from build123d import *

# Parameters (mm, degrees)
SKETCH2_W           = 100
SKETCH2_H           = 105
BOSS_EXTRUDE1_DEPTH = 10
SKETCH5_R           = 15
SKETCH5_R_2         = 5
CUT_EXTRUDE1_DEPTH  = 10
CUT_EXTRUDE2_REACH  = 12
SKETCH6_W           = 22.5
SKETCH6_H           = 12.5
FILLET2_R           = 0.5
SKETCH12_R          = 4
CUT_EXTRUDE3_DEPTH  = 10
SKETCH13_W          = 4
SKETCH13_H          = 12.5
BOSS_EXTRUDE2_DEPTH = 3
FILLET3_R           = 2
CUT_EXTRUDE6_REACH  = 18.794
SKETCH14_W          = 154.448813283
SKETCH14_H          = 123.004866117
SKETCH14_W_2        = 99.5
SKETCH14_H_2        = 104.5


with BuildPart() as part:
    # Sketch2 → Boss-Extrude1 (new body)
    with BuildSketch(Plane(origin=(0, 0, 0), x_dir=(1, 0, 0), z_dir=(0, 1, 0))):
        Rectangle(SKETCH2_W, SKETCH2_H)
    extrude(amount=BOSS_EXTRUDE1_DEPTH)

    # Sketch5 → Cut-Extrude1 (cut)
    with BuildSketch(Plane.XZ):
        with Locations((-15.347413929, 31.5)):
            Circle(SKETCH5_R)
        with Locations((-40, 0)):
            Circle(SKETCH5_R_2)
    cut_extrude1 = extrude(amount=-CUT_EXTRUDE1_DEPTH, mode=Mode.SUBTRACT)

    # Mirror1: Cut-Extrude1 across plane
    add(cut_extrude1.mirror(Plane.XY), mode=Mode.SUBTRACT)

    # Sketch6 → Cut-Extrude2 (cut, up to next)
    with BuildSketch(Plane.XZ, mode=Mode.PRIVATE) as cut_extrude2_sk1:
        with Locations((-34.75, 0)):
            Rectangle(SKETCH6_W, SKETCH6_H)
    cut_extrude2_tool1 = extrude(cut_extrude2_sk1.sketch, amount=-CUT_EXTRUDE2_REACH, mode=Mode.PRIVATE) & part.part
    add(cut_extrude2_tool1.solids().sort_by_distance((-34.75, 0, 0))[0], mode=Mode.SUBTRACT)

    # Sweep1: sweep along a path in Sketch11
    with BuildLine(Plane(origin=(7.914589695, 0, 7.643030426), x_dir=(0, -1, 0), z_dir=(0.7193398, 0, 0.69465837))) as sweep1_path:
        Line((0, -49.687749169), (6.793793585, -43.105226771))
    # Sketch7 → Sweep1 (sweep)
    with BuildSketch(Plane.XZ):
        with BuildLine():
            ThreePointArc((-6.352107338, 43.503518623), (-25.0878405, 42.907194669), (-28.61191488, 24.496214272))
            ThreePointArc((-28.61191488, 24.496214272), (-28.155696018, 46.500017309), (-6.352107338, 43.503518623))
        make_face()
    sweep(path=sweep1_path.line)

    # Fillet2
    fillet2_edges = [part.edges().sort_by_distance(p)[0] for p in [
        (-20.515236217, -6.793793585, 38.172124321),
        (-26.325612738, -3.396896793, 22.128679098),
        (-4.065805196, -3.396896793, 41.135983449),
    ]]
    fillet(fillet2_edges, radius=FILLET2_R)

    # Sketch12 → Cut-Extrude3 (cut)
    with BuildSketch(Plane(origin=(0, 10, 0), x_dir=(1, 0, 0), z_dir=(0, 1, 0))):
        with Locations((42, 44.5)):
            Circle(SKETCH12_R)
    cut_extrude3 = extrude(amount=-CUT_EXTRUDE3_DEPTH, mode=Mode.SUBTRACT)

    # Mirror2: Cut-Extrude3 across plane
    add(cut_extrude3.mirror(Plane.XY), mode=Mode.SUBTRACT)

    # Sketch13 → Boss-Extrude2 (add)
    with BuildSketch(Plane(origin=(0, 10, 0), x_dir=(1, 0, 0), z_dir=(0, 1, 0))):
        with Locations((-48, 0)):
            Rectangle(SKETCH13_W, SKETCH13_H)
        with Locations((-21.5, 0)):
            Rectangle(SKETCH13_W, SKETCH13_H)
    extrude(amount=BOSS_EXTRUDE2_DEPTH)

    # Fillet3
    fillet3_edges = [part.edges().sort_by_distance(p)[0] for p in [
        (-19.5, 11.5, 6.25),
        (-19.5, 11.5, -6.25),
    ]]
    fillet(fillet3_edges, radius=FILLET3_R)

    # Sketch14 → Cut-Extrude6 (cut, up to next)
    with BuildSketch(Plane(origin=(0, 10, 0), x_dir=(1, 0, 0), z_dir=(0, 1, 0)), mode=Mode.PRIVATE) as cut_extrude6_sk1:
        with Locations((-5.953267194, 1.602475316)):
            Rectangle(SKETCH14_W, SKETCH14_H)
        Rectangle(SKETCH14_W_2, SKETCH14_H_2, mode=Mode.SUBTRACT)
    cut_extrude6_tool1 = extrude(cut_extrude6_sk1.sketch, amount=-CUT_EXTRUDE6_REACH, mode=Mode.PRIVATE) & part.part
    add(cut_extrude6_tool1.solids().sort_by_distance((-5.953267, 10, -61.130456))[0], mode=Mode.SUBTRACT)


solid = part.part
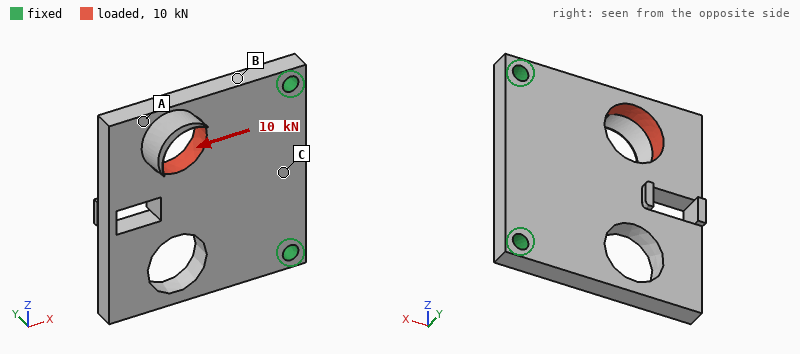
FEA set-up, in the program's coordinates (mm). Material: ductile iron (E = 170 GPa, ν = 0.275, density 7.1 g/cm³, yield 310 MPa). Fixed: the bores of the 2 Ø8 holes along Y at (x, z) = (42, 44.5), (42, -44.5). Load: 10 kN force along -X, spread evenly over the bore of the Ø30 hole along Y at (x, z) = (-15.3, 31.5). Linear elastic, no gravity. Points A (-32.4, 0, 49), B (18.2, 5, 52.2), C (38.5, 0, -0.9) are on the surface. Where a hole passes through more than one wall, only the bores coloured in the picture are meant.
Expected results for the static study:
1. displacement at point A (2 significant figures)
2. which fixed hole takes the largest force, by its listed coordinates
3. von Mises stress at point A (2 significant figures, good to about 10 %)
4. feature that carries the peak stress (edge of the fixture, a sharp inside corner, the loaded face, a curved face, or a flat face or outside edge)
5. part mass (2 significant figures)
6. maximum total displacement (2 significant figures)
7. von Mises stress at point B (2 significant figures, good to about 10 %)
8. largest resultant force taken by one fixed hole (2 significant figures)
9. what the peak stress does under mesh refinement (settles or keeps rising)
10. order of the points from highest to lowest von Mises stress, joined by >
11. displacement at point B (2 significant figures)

17 µm
(42, 44.5)
13 MPa
a sharp inside corner
620 g
20 µm
43 MPa
8.7 kN
keeps rising
B > A > C
5.5 µm
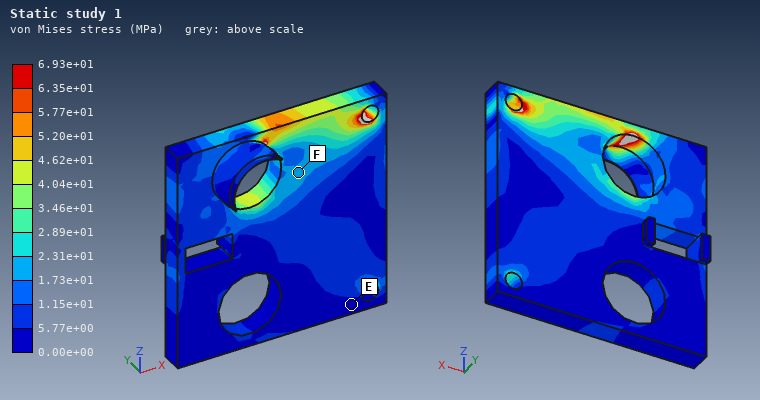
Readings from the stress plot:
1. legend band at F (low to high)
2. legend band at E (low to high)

1.73e+01 to 2.31e+01 MPa
0.00e+00 to 5.77e+00 MPa
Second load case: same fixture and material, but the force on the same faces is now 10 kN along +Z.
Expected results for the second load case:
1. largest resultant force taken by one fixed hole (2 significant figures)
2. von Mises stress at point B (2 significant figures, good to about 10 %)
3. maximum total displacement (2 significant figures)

8.1 kN
28 MPa
35 µm
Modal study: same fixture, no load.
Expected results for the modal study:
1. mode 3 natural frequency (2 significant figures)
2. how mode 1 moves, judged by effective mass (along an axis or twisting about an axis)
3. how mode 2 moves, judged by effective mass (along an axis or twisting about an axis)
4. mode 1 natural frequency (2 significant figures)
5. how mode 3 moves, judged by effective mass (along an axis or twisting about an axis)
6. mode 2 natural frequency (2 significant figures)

3900 Hz
along Y
twisting about X
820 Hz
along Y
1900 Hz
